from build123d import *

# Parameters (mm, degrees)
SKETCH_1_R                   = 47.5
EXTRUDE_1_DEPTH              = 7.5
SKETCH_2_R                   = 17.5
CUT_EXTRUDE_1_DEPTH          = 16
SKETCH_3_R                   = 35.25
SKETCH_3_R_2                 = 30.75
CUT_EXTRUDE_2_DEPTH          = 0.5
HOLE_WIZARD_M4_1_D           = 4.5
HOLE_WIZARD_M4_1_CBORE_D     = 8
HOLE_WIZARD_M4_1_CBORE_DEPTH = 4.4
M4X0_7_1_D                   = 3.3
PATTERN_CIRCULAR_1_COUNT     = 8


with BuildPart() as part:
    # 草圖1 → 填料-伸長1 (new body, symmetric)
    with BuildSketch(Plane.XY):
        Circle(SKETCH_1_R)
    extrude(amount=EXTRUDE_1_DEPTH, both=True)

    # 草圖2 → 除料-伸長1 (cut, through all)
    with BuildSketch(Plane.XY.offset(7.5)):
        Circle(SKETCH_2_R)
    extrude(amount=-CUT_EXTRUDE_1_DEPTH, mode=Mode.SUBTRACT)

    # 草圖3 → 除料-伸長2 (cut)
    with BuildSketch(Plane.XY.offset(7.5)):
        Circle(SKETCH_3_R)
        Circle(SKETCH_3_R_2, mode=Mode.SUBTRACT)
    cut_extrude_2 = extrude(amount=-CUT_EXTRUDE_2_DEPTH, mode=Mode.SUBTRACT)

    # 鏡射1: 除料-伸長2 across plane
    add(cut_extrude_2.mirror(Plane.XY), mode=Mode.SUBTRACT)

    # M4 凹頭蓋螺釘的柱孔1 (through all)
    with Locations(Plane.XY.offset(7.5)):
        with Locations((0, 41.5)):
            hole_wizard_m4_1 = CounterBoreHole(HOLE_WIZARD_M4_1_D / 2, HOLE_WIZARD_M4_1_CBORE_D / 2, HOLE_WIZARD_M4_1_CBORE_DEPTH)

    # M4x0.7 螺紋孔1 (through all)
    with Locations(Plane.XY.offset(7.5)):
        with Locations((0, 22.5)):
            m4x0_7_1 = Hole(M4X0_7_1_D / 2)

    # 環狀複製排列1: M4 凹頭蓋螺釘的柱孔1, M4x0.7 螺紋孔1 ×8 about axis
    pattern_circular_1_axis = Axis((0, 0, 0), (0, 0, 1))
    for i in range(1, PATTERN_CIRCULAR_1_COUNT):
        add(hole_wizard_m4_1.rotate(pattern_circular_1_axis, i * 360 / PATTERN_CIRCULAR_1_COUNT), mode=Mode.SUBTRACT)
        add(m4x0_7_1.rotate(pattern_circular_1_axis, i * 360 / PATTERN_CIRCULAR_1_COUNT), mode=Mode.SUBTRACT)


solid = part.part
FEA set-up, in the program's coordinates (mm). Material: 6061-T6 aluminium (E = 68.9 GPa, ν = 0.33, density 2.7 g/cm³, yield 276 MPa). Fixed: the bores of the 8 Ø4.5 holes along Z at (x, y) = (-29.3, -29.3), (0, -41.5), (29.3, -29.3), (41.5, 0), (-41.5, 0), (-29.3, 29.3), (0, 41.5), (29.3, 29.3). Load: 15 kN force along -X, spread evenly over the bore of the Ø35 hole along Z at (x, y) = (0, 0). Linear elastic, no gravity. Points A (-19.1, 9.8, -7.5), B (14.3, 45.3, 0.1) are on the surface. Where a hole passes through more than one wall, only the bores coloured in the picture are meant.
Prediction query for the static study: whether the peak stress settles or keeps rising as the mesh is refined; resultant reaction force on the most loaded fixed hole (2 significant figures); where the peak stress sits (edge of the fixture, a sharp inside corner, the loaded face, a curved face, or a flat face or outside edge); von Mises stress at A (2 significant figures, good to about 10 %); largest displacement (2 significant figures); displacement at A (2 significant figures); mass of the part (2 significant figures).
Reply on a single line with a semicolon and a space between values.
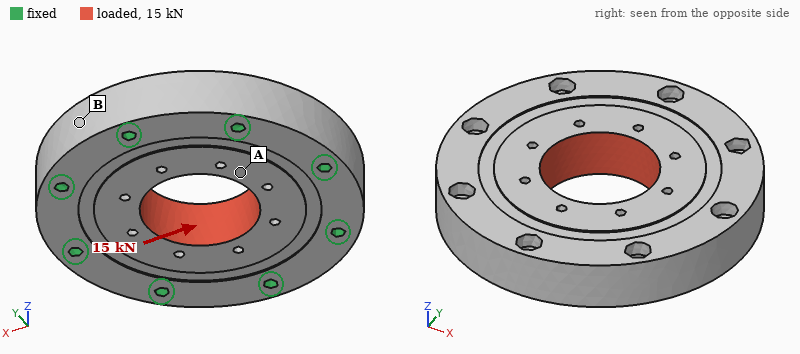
keeps rising; 2.8 kN; edge of the fixture; 8.6 MPa; 5.7 µm; 3.8 µm; 230 g
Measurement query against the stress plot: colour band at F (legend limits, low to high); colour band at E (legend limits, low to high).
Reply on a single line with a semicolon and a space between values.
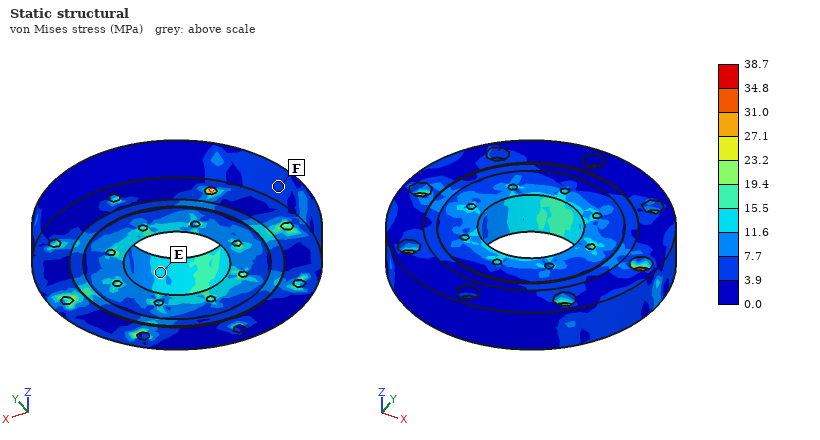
3.9 to 7.7 MPa; 11.6 to 15.5 MPa
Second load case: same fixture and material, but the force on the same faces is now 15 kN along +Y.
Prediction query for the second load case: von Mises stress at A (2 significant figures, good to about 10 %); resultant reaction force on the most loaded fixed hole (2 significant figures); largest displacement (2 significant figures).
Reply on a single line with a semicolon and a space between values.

12 MPa; 2.8 kN; 5.6 µm
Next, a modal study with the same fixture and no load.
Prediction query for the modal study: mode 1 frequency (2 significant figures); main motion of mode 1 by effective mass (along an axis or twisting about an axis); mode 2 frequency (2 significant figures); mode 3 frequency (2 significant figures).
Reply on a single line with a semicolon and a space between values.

15 kHz; along Z; 20 kHz; 21 kHz
